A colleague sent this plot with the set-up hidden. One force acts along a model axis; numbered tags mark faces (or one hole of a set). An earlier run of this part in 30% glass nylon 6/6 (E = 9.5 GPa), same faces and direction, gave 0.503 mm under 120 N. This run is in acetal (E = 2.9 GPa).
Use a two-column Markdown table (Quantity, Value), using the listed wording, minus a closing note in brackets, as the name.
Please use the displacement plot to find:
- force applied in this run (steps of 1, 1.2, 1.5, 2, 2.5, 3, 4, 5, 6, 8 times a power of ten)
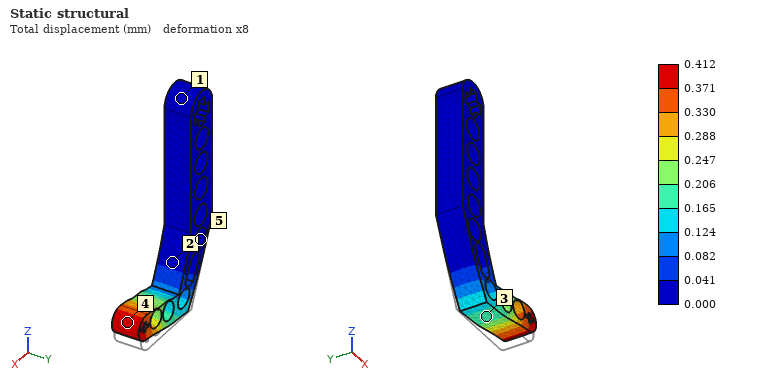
| Quantity | Value |
|---|---|
| force applied in this run | 30 N |
